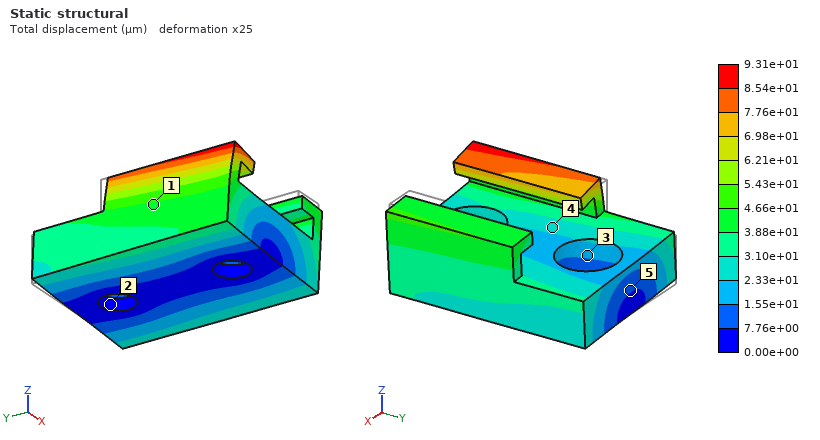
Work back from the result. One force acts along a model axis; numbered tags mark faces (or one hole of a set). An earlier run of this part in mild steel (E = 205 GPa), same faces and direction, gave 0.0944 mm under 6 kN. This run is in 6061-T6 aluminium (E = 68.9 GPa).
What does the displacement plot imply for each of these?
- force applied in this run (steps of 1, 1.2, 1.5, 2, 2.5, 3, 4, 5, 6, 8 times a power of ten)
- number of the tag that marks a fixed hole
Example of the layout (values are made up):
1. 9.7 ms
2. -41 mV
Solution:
1. 2 kN
2. 2
